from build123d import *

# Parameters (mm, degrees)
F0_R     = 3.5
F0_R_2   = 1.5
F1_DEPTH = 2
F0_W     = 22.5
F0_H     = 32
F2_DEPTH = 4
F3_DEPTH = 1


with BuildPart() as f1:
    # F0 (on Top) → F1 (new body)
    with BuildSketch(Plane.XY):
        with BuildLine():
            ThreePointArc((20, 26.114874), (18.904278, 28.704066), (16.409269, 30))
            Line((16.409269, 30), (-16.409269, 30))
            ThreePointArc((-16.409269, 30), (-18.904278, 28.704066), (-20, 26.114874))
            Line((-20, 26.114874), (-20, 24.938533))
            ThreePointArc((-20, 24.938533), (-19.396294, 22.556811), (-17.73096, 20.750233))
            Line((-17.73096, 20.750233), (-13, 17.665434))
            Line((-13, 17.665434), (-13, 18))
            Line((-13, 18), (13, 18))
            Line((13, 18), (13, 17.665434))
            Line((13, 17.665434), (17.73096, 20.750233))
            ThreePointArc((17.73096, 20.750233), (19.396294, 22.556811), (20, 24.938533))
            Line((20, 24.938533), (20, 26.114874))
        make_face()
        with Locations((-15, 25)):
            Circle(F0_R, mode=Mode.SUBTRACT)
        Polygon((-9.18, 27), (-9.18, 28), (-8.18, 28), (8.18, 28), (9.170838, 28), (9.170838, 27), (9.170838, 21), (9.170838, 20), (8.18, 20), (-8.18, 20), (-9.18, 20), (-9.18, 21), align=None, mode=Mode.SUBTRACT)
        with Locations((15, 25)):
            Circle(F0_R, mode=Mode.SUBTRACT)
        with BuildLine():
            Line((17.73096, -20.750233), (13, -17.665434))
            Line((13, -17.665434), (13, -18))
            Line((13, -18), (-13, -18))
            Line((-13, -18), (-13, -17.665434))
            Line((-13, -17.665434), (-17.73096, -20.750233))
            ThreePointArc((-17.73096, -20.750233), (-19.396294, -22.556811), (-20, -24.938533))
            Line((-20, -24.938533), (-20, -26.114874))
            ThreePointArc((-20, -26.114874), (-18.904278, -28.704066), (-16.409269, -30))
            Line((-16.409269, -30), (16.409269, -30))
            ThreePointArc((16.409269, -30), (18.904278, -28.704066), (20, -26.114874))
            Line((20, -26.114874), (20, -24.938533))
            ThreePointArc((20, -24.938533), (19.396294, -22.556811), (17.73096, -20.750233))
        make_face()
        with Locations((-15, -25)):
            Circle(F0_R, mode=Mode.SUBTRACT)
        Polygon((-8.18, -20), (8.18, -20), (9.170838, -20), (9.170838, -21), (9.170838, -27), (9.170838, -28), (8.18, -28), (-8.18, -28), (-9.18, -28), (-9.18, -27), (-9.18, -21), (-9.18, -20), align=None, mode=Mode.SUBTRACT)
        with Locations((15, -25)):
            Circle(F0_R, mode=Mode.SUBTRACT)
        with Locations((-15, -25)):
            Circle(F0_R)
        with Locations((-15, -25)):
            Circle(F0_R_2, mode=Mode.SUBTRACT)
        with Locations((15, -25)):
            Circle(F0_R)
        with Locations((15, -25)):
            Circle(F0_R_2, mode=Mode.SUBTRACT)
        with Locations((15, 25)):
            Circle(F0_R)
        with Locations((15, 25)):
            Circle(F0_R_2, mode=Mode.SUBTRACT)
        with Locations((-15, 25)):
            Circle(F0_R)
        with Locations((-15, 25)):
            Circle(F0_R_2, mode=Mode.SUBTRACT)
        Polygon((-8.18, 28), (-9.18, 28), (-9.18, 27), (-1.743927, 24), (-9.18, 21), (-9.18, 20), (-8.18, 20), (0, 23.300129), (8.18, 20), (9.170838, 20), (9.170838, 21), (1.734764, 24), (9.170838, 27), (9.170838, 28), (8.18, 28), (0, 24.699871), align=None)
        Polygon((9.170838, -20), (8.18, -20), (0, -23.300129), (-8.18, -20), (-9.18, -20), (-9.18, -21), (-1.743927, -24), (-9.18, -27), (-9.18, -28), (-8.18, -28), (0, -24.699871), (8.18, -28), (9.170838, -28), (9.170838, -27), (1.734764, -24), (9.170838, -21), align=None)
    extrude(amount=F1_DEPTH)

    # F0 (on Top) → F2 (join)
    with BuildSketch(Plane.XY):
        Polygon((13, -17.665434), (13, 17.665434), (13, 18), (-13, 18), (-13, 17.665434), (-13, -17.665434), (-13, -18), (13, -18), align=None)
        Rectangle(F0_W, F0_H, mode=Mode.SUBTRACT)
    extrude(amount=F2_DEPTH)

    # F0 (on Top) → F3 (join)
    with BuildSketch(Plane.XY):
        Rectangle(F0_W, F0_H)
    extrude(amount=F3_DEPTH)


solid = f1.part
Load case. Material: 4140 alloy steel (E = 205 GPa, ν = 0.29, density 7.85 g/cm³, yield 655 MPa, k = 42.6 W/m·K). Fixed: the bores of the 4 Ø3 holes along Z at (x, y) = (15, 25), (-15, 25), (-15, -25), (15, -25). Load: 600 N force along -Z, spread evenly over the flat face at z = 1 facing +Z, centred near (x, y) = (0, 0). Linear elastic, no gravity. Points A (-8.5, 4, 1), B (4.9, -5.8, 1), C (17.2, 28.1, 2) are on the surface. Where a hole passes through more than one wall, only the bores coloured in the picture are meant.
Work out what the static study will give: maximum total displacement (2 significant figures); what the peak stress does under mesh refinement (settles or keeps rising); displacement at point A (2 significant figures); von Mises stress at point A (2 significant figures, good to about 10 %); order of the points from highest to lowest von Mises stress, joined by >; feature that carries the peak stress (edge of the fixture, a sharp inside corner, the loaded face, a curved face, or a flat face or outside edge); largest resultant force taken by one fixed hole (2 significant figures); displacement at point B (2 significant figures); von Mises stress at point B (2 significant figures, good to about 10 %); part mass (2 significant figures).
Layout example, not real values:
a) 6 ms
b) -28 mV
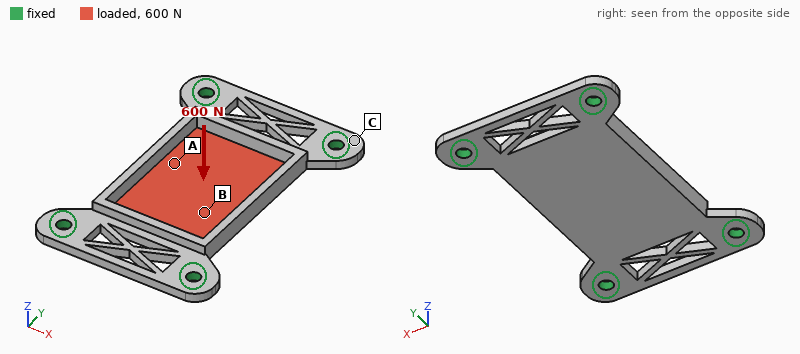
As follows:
a) 0.12 mm
b) keeps rising
c) 0.081 mm
d) 44 MPa
e) B > A > C
f) edge of the fixture
g) 160 N
h) 0.093 mm
i) 81 MPa
j) 23 g
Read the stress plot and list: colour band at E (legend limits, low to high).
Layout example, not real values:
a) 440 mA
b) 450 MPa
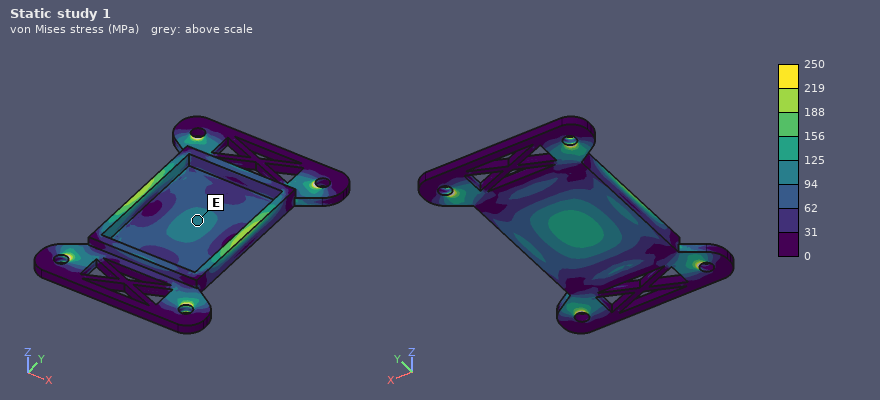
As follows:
a) 94 to 125 MPa
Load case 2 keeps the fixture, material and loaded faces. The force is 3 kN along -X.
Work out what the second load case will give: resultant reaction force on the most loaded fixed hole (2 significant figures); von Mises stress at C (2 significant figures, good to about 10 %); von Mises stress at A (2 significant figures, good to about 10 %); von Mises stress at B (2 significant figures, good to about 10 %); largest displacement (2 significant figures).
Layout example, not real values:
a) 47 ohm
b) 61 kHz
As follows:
a) 980 N
b) 17 MPa
c) 31 MPa
d) 56 MPa
e) 23 µm
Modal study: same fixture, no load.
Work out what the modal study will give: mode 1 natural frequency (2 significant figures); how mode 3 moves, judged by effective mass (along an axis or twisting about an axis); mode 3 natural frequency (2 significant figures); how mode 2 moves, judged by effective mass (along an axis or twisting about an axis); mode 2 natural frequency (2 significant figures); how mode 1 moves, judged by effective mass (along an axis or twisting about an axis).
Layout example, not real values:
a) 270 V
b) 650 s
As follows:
a) 4800 Hz
b) twisting about X
c) 10 kHz
d) twisting about Y
e) 7700 Hz
f) along Z
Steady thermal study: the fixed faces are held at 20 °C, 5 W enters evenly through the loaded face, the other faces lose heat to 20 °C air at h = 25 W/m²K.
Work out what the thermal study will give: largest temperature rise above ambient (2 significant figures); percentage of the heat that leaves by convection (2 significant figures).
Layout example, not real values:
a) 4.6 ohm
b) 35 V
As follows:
a) 29 K
b) 24 %
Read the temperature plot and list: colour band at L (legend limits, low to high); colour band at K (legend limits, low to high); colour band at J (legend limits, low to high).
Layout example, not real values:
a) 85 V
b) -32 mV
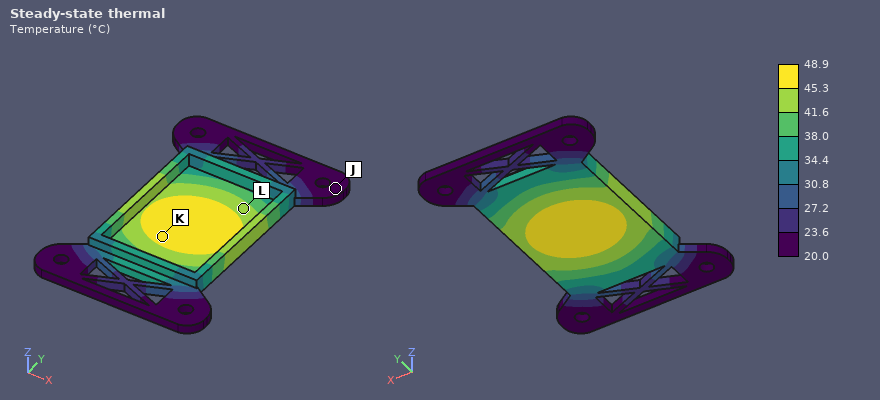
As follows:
a) 41.6 to 45.3 °C
b) 45.3 to 48.9 °C
c) 20.0 to 23.6 °C
